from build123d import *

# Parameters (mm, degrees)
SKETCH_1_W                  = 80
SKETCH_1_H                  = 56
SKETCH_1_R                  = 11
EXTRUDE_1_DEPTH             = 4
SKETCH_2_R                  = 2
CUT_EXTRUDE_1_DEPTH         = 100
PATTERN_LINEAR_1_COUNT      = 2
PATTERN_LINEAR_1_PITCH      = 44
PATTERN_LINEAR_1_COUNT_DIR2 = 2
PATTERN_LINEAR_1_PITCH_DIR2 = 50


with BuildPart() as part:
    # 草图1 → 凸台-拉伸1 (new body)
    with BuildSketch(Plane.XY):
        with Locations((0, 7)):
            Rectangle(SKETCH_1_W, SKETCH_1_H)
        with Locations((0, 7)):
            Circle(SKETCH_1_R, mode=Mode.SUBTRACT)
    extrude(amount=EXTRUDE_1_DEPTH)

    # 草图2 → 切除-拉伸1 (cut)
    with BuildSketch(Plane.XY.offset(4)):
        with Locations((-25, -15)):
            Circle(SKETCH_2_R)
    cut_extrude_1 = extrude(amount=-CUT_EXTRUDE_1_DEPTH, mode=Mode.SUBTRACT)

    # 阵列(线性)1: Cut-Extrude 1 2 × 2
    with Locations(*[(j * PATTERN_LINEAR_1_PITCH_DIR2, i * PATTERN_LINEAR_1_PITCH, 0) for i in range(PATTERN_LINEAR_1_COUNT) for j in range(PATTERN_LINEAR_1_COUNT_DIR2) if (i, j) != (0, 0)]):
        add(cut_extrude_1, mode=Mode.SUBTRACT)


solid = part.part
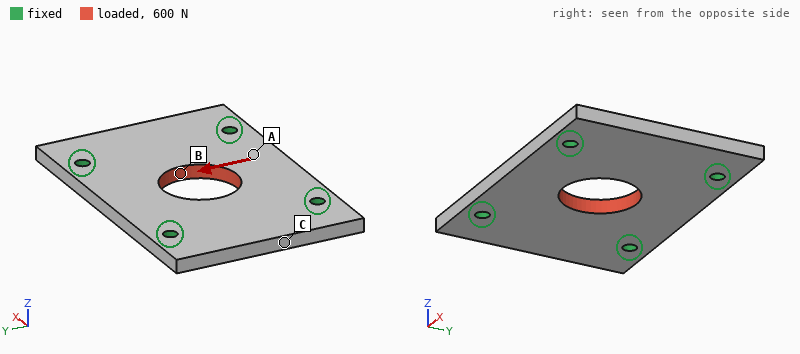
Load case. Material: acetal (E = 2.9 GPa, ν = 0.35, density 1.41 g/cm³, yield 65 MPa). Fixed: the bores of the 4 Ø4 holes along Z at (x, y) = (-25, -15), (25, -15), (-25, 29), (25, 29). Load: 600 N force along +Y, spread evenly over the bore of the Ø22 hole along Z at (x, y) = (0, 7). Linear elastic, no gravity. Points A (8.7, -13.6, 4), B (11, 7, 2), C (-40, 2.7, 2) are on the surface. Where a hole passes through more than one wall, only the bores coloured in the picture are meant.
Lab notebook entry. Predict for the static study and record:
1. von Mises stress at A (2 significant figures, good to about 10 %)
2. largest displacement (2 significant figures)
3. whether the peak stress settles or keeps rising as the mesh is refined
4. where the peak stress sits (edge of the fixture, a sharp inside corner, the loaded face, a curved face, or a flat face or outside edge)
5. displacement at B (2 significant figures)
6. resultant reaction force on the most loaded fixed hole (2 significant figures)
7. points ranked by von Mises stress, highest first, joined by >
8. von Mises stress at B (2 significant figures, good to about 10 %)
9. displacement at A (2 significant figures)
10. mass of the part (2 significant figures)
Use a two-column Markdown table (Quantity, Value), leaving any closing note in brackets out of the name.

| Quantity | Value |
|---|---|
| von Mises stress at A | 1.7 MPa |
| largest displacement | 39 µm |
| whether the peak stress settles or keeps rising as the mesh is refined | keeps rising |
| where the peak stress sits | edge of the fixture |
| displacement at B | 27 µm |
| resultant reaction force on the most loaded fixed hole | 170 N |
| points ranked by von Mises stress, highest first, joined by > | B > A > C |
| von Mises stress at B | 3.8 MPa |
| displacement at A | 28 µm |
| mass of the part | 23 g |
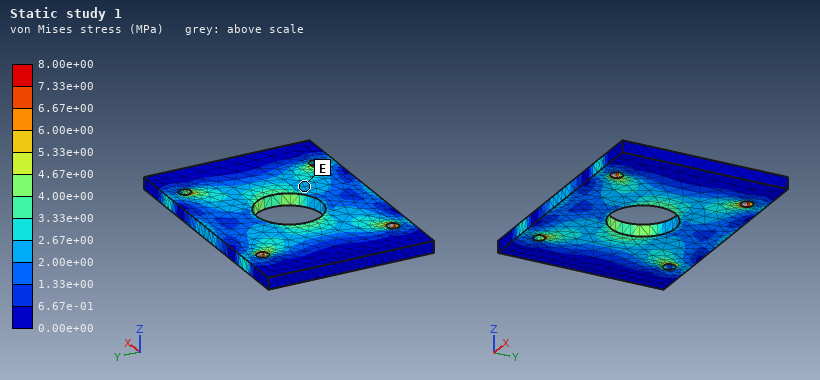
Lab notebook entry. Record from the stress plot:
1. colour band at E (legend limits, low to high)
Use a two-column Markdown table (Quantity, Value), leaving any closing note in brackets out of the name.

| Quantity | Value |
|---|---|
| colour band at E | 2.00e+00 to 2.67e+00 MPa |
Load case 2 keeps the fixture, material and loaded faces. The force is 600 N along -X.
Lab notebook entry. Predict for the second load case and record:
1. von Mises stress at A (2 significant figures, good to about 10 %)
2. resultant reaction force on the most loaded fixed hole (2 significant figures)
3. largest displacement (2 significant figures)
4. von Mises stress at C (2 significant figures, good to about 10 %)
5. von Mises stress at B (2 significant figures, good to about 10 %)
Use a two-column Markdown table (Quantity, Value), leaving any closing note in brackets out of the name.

| Quantity | Value |
|---|---|
| von Mises stress at A | 1.3 MPa |
| resultant reaction force on the most loaded fixed hole | 150 N |
| largest displacement | 26 µm |
| von Mises stress at C | 1.7 MPa |
| von Mises stress at B | 2.1 MPa |
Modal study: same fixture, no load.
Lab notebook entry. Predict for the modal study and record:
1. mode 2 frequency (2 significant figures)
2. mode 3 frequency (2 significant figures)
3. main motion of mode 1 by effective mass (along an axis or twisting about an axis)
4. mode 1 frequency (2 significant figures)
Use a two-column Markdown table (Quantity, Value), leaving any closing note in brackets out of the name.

| Quantity | Value |
|---|---|
| mode 2 frequency | 2400 Hz |
| mode 3 frequency | 2400 Hz |
| main motion of mode 1 by effective mass | along Z |
| mode 1 frequency | 2000 Hz |
